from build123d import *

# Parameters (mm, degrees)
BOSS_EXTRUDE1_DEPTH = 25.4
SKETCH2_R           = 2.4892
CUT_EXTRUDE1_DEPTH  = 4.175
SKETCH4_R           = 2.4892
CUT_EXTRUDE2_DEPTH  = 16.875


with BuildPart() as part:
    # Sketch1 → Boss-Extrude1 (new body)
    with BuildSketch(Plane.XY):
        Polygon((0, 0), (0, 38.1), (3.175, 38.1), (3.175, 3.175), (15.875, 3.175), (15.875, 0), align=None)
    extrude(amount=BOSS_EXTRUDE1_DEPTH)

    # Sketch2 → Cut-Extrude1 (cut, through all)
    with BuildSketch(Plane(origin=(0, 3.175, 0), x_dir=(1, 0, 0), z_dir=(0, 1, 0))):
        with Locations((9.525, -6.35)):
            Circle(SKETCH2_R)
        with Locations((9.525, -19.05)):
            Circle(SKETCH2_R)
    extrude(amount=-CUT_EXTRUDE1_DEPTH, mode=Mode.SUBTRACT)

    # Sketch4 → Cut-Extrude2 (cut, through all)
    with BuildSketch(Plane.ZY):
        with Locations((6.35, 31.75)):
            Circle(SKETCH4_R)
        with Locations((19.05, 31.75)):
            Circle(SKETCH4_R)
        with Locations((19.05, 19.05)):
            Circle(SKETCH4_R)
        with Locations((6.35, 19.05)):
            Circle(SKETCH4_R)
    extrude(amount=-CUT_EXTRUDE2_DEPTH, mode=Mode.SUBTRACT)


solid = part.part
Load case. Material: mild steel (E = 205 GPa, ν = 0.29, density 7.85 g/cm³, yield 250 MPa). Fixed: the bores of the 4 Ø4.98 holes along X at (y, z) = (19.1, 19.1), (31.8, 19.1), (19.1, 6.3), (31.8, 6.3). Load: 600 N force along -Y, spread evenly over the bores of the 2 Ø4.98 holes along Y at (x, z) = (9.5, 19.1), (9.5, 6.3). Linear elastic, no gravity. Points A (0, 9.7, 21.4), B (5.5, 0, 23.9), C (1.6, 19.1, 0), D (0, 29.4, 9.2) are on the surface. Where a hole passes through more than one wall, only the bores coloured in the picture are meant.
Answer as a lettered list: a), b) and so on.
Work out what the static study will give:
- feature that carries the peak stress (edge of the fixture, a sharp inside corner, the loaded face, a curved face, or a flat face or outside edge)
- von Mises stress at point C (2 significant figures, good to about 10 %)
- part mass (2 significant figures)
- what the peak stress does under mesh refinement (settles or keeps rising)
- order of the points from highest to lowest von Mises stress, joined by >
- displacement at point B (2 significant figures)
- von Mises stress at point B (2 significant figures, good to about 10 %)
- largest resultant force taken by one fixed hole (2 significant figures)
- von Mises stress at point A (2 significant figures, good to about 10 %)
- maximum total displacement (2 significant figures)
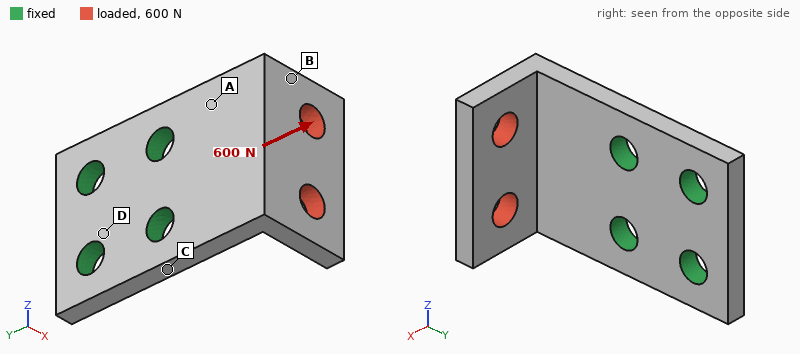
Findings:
a) edge of the fixture
b) 25 MPa
c) 29 g
d) keeps rising
e) A > B > C > D
f) 0.055 mm
g) 62 MPa
h) 280 N
i) 98 MPa
j) 0.10 mm
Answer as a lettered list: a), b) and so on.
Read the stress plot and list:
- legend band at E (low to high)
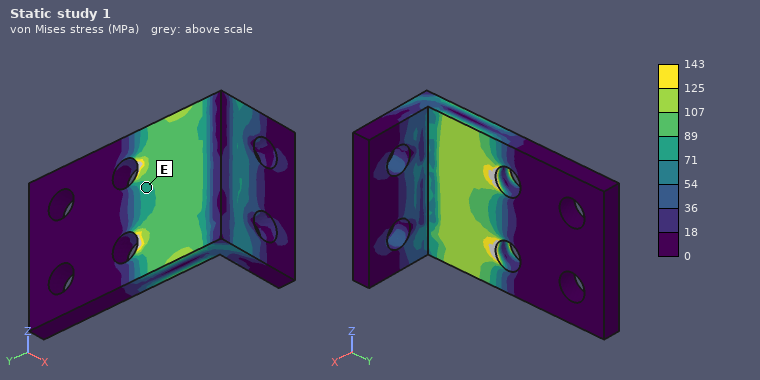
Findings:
a) 71 to 89 MPa
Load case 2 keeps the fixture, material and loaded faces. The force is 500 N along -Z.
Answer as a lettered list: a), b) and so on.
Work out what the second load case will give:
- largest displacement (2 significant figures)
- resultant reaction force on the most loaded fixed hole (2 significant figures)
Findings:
a) 34 µm
b) 560 N
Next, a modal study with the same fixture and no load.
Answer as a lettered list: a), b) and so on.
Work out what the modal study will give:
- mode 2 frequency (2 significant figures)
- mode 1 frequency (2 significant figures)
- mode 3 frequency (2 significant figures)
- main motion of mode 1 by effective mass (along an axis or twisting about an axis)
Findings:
a) 7000 Hz
b) 4000 Hz
c) 11 kHz
d) along X
